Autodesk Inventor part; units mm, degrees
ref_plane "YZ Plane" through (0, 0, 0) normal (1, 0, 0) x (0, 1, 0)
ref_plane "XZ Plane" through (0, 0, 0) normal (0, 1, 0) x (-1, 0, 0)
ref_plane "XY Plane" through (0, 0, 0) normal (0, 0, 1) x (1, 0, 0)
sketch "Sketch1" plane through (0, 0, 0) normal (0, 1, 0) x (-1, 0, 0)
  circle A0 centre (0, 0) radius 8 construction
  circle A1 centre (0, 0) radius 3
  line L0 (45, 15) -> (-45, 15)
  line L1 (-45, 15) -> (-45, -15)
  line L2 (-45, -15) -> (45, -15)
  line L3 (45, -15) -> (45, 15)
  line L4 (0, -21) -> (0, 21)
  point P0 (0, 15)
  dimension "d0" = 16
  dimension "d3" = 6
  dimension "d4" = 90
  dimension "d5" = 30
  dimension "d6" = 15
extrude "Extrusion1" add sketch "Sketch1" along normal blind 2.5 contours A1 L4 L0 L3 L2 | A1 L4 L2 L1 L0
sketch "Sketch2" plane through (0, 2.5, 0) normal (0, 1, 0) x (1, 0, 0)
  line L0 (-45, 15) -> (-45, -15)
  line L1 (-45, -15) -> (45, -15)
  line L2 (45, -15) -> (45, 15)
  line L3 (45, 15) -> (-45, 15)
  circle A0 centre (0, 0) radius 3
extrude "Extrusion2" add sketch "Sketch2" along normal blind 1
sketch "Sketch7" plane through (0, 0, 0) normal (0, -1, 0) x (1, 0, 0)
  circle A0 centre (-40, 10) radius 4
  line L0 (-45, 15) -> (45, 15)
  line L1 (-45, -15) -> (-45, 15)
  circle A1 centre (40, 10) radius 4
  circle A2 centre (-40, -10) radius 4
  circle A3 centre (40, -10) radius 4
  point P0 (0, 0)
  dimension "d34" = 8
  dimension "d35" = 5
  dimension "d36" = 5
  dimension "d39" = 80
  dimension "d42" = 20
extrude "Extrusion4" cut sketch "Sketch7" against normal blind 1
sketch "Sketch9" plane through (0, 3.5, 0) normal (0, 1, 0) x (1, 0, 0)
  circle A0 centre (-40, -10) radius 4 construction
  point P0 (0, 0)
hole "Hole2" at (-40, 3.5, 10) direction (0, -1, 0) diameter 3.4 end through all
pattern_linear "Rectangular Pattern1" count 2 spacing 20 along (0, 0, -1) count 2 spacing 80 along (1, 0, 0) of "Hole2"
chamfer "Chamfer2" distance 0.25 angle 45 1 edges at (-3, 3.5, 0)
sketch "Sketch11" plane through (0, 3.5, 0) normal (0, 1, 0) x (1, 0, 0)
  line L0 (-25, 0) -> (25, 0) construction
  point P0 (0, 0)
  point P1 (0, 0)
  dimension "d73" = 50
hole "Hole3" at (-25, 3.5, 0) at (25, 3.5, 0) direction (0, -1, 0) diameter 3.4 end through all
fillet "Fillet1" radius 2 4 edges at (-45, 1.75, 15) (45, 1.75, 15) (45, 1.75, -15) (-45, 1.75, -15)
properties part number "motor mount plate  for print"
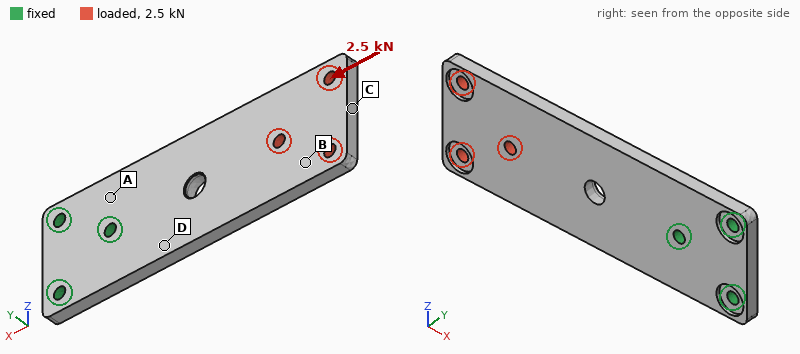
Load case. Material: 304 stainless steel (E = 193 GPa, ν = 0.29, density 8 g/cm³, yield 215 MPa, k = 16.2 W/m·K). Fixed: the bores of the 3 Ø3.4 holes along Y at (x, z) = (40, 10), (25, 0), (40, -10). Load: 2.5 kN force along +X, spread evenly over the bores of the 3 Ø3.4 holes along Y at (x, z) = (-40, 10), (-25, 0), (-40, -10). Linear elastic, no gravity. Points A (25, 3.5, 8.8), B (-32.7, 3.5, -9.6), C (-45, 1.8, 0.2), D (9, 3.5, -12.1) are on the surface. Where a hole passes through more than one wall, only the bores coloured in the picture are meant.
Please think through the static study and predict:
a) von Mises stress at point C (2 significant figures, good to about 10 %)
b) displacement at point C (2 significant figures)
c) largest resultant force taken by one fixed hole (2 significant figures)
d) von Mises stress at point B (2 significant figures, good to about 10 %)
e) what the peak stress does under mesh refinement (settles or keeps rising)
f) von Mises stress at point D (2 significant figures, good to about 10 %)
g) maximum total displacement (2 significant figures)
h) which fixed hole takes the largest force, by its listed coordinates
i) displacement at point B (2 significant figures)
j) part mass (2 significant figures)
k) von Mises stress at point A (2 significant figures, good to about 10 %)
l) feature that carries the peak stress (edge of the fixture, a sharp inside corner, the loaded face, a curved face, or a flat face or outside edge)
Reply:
12 MPa
92 µm
1.6 kN
31 MPa
keeps rising
37 MPa
93 µm
(25, 0)
64 µm
72 g
24 MPa
edge of the fixture
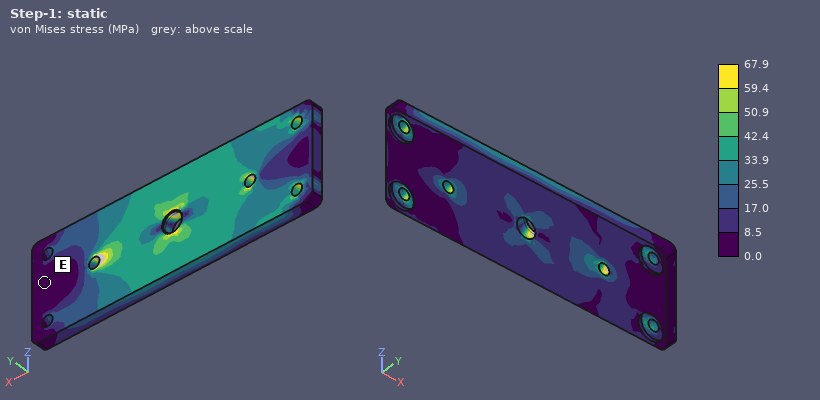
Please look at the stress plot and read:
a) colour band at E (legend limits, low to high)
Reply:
0.0 to 8.5 MPa
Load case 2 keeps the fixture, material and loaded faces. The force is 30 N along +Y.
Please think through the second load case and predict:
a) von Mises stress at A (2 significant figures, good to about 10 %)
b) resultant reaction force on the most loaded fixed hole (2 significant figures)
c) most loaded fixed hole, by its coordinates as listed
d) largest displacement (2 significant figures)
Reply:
16 MPa
90 N
(25, 0)
0.13 mm
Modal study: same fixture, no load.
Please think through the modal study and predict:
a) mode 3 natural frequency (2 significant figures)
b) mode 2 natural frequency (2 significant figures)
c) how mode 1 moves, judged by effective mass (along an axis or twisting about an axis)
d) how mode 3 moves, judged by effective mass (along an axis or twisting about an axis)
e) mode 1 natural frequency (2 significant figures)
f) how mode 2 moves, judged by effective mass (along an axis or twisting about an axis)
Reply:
3400 Hz
2400 Hz
along Y
along Y
570 Hz
twisting about X
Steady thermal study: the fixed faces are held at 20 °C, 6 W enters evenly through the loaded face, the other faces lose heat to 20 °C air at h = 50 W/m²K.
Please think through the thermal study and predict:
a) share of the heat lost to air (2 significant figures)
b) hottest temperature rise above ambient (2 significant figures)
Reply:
92 %
57 K
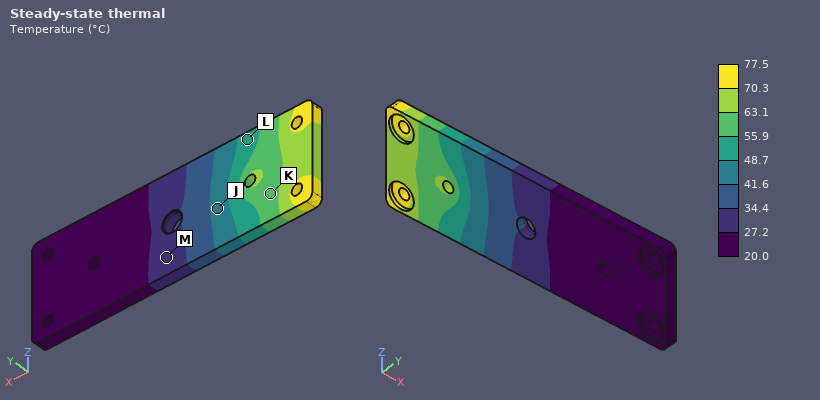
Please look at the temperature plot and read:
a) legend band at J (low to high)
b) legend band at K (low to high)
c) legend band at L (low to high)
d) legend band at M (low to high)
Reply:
41.6 to 48.7 °C
55.9 to 63.1 °C
48.7 to 55.9 °C
27.2 to 34.4 °C
